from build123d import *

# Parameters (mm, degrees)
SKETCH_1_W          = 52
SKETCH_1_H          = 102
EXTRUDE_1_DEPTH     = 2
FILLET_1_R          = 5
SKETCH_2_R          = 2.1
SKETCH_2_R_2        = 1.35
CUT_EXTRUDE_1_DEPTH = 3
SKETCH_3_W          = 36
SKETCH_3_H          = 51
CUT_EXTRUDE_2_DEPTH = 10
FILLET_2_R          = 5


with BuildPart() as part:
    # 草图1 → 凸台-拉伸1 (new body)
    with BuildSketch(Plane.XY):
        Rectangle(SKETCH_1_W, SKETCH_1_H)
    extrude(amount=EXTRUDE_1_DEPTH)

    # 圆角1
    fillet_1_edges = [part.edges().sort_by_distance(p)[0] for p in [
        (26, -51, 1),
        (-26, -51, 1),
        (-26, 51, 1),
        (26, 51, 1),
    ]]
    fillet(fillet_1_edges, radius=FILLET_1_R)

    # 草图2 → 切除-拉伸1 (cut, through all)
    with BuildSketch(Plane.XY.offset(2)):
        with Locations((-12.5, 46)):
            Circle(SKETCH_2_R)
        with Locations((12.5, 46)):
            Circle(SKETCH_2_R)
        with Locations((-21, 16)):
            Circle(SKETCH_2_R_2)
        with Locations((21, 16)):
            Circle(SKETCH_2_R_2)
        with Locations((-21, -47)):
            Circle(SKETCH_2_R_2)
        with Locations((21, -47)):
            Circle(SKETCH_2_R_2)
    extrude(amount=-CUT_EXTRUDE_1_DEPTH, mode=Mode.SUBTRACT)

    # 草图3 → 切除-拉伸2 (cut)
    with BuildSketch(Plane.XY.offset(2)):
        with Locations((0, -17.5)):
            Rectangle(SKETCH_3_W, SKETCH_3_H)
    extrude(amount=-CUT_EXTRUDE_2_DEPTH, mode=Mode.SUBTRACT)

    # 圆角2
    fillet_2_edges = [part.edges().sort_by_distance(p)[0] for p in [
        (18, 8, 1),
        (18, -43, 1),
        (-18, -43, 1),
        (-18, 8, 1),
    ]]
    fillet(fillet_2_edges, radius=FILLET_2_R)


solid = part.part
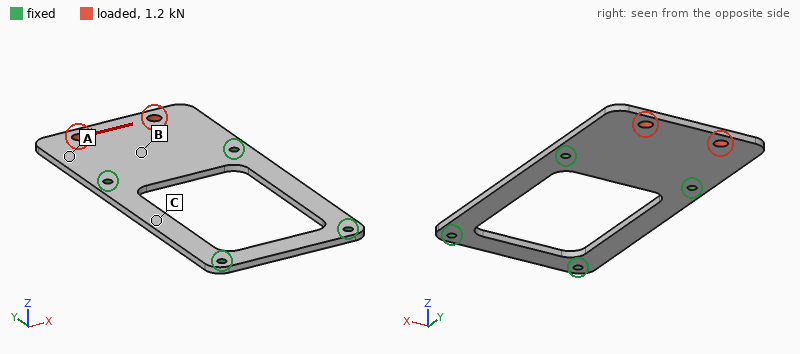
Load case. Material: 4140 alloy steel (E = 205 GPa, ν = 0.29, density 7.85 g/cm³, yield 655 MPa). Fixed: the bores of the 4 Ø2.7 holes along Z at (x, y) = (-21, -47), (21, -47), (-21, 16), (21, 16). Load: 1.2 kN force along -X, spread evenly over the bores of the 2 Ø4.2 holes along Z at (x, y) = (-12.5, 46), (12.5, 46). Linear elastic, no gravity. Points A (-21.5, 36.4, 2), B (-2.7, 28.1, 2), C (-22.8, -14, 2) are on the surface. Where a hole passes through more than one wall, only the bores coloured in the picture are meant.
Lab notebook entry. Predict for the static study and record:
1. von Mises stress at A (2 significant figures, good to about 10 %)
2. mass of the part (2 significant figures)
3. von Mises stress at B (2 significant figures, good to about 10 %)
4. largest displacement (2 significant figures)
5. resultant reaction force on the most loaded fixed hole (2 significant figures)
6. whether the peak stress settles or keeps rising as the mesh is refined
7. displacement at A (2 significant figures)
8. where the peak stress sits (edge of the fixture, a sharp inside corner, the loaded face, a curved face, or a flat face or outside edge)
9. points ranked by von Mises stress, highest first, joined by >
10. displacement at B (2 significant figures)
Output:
15 MPa
54 g
25 MPa
10 µm
1.0 kN
keeps rising
6.3 µm
edge of the fixture
B > A > C
3.4 µm
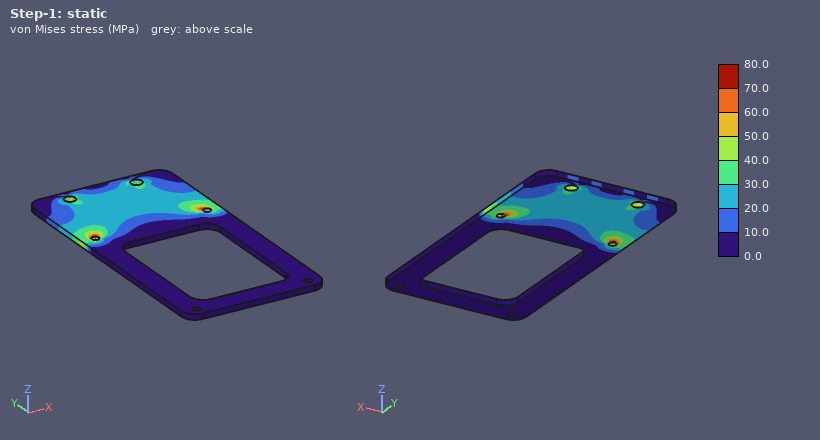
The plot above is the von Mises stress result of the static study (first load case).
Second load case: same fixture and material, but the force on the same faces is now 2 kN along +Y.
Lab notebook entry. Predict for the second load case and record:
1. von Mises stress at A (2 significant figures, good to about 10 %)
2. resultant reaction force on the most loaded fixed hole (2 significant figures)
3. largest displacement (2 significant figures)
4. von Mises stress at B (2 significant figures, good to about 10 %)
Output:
21 MPa
1.0 kN
6.6 µm
9.9 MPa
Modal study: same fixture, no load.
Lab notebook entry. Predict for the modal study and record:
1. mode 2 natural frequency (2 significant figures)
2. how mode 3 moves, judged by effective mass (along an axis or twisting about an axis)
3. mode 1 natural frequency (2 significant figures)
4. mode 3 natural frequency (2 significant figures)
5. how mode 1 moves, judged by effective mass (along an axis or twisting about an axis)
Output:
2600 Hz
along Z
1200 Hz
3000 Hz
along Z
